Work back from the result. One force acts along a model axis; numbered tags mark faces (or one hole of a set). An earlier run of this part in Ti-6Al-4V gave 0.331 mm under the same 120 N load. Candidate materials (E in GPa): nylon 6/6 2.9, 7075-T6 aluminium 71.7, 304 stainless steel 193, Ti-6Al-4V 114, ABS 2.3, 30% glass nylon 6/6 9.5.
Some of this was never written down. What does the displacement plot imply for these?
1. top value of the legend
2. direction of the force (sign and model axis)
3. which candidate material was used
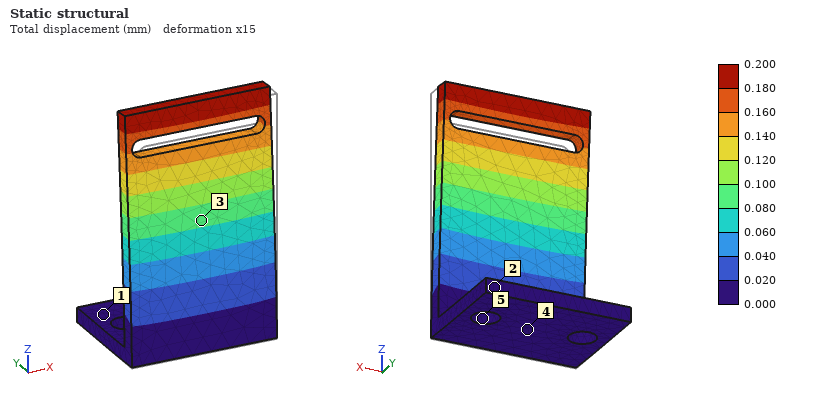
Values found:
0.200 mm
+Y
304 stainless steel
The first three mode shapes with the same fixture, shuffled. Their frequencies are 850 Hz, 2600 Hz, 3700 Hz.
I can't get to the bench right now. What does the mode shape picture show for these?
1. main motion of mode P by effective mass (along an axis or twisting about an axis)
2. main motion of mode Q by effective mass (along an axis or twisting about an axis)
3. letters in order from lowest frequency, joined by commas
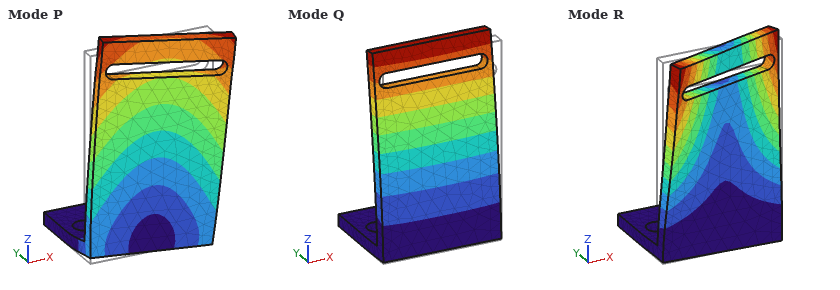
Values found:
along X
along Y
Q, P, R
